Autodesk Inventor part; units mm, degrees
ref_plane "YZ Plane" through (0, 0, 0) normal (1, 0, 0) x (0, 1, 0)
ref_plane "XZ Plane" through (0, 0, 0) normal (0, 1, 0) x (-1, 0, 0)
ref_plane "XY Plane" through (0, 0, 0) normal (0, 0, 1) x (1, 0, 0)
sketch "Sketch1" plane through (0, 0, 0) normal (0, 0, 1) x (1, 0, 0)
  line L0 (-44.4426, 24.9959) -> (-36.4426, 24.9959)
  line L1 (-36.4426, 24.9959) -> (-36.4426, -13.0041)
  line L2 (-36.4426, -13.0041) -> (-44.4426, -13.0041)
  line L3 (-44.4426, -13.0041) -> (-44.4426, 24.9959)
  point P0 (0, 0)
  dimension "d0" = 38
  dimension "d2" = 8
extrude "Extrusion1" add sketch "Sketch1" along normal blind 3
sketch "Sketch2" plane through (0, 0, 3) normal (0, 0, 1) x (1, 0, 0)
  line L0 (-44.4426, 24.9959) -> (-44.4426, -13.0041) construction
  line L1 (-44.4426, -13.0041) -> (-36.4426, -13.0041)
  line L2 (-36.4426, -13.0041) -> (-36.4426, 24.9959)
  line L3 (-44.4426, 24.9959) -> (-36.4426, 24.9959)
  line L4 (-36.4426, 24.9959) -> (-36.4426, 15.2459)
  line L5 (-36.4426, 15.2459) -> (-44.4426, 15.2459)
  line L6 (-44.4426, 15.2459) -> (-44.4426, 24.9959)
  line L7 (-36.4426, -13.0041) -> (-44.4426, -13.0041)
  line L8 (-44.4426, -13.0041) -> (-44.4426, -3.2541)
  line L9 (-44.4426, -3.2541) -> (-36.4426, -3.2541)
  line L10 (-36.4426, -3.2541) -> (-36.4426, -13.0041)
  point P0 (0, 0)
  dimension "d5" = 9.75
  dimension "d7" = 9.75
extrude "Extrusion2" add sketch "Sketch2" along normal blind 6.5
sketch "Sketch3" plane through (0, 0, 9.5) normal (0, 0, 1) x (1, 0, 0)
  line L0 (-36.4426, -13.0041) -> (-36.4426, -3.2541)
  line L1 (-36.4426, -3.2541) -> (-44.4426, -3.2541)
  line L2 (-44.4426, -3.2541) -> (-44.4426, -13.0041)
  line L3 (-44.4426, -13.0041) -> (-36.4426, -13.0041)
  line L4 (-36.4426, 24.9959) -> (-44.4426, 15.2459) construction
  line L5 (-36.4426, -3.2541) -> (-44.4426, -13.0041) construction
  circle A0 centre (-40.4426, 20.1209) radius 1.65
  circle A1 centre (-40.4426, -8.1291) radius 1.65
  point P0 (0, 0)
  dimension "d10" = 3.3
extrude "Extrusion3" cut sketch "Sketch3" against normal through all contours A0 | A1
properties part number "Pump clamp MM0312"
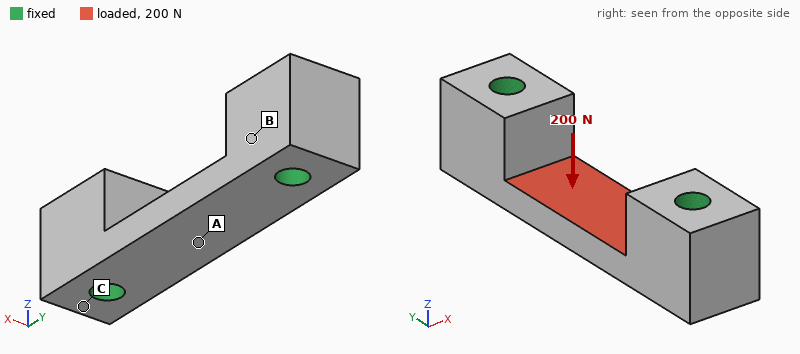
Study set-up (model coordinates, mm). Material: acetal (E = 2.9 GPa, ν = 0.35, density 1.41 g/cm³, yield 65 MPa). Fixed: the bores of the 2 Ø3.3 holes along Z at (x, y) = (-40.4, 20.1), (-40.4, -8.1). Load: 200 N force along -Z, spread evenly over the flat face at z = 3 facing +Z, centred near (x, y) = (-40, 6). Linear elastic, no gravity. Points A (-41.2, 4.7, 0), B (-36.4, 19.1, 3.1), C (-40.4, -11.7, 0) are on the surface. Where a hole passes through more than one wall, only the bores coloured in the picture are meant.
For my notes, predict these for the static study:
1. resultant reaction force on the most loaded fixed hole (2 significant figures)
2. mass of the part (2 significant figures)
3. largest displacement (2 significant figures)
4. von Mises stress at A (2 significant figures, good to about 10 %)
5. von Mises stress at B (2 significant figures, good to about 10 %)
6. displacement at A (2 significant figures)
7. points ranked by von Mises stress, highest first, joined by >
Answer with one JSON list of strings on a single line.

["100 N", "2.5 g", "0.15 mm", "17 MPa", "3.3 MPa", "0.13 mm", "A > B > C"]
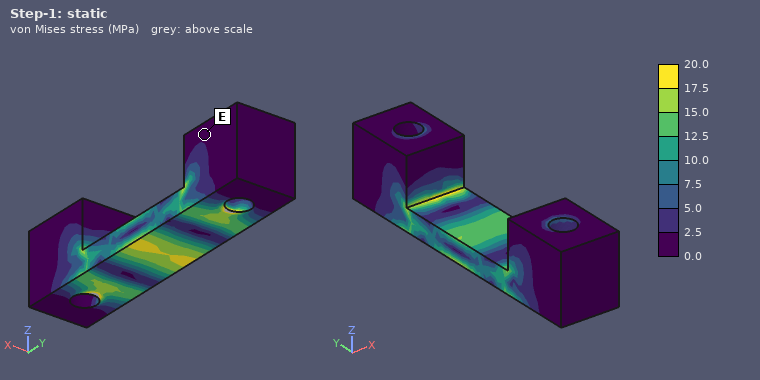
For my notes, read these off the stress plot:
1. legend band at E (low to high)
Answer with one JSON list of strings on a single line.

["0.0 to 2.5 MPa"]
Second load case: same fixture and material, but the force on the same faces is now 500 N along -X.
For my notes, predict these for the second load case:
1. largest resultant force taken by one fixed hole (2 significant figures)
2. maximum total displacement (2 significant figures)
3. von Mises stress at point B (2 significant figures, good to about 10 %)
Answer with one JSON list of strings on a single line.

["250 N", "0.26 mm", "13 MPa"]
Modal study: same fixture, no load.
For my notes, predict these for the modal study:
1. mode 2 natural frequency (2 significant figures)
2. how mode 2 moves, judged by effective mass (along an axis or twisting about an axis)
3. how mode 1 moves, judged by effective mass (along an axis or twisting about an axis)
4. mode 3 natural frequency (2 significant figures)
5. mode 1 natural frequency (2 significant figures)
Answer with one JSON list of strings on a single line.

["11 kHz", "along X", "along Z", "14 kHz", "8500 Hz"]
